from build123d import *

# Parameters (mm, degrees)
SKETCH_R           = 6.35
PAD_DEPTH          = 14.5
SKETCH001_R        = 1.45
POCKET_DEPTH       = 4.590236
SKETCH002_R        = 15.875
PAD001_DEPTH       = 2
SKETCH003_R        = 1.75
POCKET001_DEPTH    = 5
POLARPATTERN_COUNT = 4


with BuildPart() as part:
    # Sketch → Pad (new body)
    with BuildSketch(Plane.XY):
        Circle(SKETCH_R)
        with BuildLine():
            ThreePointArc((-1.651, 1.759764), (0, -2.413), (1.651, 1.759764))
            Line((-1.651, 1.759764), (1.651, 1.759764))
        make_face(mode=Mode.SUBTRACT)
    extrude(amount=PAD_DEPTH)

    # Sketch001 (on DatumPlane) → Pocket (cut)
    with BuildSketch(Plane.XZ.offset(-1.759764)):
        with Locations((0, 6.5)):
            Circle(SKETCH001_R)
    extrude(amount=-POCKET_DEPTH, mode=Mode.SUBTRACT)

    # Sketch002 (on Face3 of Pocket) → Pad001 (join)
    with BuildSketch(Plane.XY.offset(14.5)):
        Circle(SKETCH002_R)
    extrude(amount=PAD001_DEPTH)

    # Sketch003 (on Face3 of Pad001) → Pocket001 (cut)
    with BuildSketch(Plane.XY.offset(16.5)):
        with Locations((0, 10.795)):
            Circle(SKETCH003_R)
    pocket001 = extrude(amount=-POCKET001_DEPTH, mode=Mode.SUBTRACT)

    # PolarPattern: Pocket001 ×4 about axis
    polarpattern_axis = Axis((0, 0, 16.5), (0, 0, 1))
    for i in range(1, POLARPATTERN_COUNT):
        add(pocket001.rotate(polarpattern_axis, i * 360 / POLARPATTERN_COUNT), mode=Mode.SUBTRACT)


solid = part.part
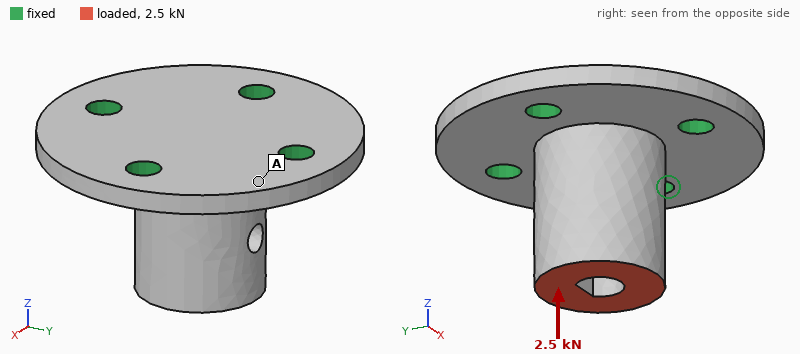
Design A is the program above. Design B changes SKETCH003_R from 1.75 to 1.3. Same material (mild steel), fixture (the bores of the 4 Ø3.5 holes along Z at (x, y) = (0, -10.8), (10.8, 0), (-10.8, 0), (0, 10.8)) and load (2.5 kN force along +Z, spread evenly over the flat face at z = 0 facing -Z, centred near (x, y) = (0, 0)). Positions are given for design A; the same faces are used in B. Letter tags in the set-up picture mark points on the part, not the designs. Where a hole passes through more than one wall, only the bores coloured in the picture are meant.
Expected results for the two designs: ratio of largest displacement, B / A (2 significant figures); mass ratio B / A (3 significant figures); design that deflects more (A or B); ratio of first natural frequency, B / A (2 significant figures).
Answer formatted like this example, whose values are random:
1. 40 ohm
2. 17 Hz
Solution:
1. 1.2
2. 1.01
3. B
4. 0.92
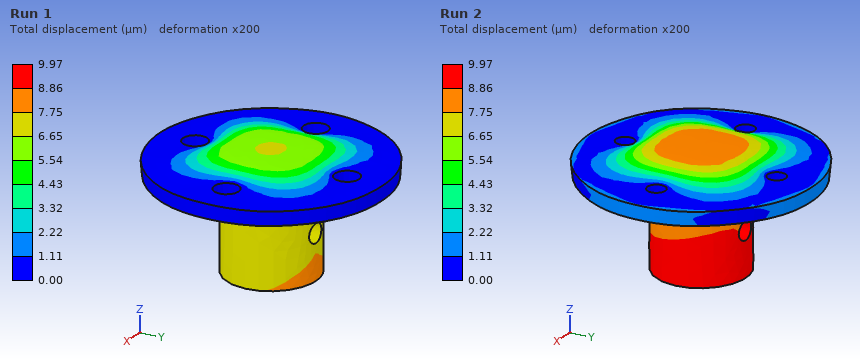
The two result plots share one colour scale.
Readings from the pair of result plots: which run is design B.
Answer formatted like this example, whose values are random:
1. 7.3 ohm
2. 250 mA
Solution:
1. Run 2
